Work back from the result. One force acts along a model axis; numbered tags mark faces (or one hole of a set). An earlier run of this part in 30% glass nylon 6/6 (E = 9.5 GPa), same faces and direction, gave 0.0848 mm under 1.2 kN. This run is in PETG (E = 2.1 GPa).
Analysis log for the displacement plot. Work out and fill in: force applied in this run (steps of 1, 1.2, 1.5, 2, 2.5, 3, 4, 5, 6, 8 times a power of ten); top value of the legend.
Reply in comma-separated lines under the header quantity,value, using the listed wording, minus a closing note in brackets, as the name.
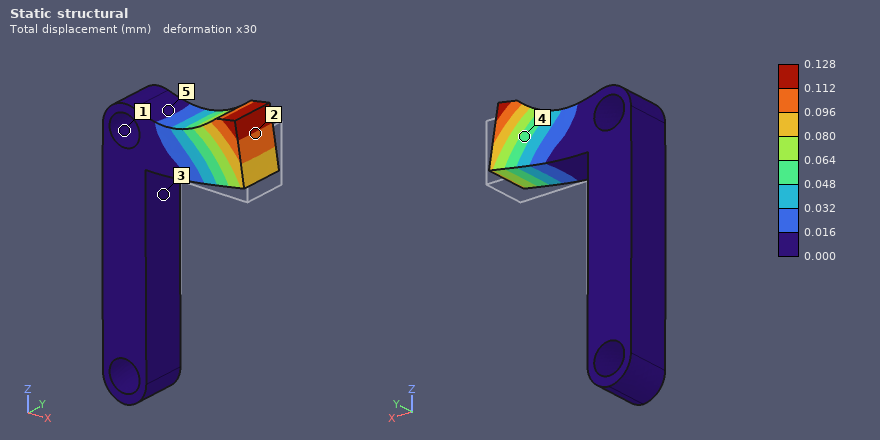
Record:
quantity,value
force applied in this run,400 N
top value of the legend,0.128 mm
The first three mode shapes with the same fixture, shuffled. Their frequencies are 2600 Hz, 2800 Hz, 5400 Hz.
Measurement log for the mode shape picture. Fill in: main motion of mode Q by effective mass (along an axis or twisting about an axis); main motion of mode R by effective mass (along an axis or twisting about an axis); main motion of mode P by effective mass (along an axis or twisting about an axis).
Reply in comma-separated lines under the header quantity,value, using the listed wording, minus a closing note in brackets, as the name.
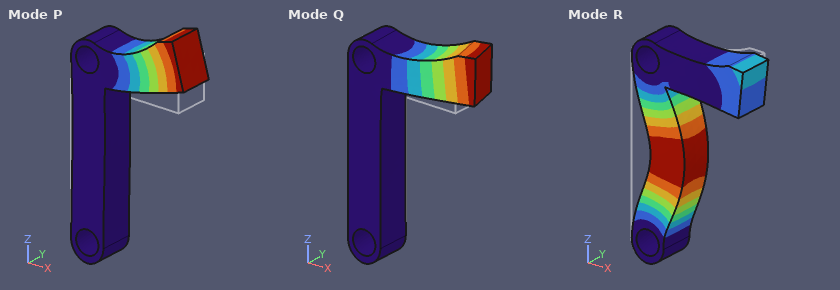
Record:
quantity,value
main motion of mode Q by effective mass,along Y
main motion of mode R by effective mass,along X
main motion of mode P by effective mass,along Z
